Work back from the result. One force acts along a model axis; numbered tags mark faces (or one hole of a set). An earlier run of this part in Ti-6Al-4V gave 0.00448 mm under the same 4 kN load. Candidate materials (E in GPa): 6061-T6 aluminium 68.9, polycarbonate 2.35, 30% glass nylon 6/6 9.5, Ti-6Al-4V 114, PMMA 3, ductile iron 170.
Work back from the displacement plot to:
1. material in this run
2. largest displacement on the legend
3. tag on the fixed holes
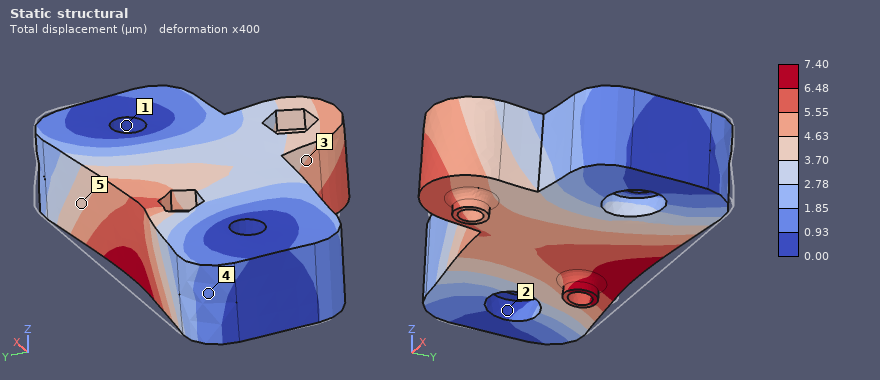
6061-T6 aluminium
7.40 µm
1
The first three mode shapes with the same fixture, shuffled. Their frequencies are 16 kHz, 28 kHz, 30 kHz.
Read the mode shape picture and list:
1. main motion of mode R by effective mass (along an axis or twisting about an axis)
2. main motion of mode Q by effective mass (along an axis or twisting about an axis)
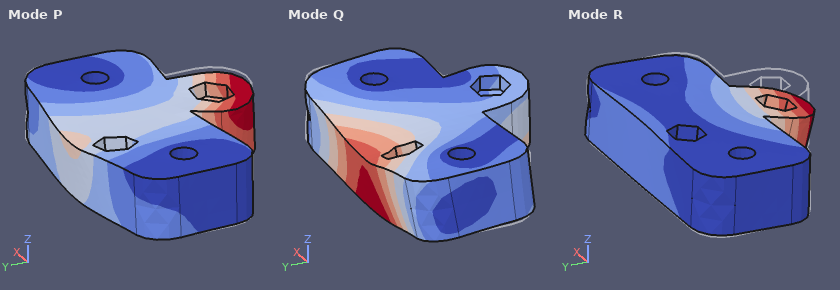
along Z
along Z
